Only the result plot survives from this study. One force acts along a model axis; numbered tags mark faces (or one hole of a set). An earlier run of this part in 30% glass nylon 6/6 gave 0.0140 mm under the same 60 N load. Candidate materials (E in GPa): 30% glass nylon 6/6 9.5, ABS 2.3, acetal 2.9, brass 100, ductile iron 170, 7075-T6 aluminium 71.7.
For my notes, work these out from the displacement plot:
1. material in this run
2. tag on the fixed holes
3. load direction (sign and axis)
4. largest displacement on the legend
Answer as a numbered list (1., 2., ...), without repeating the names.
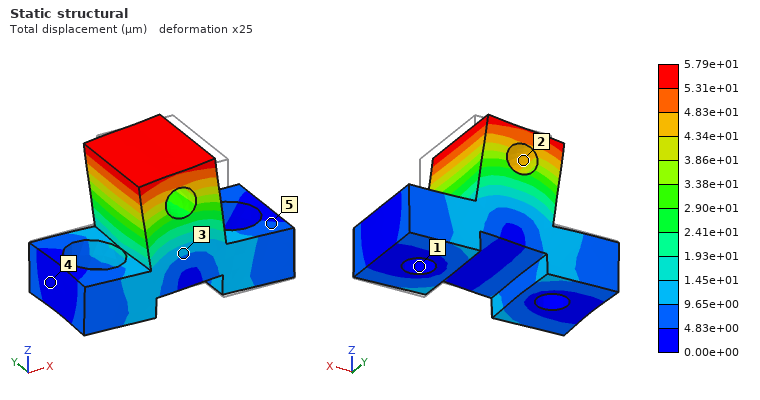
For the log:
1. ABS
2. 1
3. -X
4. 5.79e+01 µm
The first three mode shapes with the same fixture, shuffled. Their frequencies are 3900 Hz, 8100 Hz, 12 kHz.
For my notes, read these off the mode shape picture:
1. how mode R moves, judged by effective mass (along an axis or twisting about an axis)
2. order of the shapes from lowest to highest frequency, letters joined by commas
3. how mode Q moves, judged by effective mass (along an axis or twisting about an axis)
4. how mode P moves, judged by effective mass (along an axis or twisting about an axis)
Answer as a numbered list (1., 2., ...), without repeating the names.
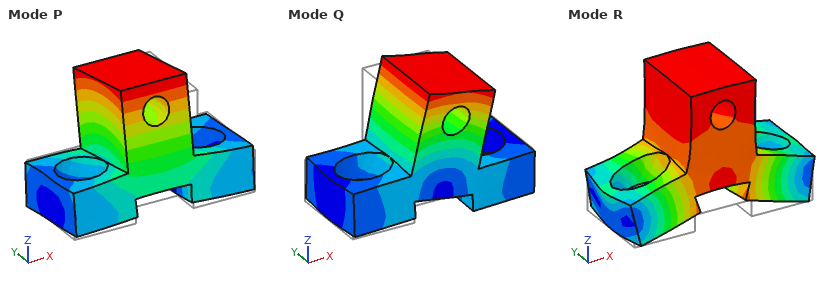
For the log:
1. along Z
2. P, Q, R
3. along X
4. along Y
